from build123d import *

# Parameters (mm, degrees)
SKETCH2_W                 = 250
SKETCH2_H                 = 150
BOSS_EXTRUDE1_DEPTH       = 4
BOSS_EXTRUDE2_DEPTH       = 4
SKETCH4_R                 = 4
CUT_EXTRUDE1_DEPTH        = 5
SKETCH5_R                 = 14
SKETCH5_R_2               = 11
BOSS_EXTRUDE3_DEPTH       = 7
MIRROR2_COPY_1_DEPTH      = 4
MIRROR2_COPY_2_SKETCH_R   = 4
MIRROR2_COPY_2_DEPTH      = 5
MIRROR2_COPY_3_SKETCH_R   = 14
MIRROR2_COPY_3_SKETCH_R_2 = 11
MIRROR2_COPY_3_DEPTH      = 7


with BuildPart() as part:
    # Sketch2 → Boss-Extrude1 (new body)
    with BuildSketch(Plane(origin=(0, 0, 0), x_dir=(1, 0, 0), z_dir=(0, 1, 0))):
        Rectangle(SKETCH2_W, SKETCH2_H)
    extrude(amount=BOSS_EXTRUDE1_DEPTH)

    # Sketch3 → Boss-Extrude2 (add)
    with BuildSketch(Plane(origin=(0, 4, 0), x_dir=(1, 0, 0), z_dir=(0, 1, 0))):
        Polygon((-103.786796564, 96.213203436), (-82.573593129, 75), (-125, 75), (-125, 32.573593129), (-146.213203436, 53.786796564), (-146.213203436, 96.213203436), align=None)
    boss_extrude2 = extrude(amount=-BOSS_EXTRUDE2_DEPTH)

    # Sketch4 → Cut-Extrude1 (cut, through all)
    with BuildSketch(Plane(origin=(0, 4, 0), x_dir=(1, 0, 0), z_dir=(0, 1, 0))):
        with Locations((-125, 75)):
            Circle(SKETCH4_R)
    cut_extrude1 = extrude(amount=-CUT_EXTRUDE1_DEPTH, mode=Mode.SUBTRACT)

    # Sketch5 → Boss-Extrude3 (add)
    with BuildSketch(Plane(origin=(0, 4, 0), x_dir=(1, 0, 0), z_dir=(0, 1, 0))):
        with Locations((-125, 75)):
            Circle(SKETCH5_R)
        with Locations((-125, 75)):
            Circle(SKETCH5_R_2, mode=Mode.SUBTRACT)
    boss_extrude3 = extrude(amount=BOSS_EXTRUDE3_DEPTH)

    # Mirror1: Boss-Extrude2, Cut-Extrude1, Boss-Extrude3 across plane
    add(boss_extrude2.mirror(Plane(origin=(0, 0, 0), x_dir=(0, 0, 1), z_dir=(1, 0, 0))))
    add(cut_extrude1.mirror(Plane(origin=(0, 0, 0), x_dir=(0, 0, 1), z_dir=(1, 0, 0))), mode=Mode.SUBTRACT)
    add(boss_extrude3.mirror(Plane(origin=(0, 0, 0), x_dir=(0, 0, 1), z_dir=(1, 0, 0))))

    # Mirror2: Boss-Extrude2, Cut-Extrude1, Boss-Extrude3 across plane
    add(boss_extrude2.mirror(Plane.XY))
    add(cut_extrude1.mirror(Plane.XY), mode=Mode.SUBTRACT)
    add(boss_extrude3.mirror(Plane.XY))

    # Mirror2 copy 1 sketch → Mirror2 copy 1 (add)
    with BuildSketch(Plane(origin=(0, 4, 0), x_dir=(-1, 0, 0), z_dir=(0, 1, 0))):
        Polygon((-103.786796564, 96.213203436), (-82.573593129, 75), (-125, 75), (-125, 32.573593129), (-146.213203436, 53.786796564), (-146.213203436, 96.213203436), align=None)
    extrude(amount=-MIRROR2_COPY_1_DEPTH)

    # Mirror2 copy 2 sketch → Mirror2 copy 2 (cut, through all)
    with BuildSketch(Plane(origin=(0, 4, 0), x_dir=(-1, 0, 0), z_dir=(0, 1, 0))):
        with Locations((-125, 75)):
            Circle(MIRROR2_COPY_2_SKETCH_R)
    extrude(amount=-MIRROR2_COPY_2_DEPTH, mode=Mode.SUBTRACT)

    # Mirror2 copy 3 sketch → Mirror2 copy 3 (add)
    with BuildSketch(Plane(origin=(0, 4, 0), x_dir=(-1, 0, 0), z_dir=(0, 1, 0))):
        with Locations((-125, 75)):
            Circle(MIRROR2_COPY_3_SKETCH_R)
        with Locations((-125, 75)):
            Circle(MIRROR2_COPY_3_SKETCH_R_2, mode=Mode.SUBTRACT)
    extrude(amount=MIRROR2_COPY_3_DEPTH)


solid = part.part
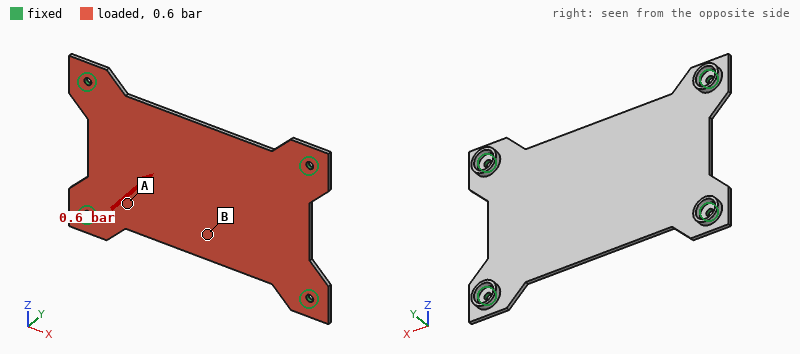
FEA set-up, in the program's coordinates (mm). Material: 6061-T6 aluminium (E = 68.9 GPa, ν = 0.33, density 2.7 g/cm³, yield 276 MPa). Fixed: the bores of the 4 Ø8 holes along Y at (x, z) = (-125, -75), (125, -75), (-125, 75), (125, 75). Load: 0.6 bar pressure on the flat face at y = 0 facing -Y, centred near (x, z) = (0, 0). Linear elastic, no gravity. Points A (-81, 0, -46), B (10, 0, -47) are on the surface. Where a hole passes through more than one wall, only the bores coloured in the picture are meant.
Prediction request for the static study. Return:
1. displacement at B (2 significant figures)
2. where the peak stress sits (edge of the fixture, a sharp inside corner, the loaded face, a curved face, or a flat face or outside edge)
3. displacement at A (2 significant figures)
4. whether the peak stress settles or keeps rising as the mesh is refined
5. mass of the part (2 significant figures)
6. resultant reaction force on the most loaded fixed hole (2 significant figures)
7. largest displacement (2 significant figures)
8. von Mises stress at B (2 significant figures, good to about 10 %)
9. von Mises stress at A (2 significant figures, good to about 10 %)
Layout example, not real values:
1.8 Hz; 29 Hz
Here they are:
1.9 mm; edge of the fixture; 0.81 mm; keeps rising; 500 g; 670 N; 2.0 mm; 59 MPa; 20 MPa
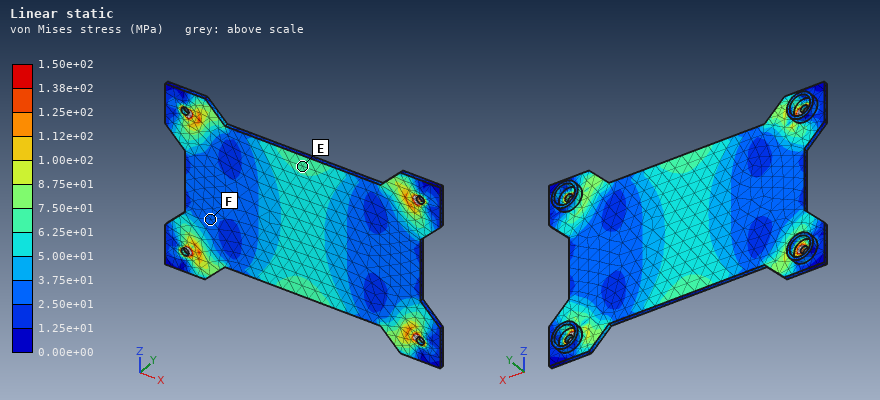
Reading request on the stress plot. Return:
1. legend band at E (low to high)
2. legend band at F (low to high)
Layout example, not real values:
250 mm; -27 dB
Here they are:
6.25e+01 to 7.50e+01 MPa; 2.50e+01 to 3.75e+01 MPa
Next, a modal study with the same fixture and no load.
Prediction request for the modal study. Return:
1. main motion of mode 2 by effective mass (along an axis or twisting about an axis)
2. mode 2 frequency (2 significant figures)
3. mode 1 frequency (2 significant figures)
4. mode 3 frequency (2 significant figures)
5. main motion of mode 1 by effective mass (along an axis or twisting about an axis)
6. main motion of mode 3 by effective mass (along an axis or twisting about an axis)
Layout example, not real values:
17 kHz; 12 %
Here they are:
twisting about X; 550 Hz; 300 Hz; 770 Hz; along Y; twisting about Z
